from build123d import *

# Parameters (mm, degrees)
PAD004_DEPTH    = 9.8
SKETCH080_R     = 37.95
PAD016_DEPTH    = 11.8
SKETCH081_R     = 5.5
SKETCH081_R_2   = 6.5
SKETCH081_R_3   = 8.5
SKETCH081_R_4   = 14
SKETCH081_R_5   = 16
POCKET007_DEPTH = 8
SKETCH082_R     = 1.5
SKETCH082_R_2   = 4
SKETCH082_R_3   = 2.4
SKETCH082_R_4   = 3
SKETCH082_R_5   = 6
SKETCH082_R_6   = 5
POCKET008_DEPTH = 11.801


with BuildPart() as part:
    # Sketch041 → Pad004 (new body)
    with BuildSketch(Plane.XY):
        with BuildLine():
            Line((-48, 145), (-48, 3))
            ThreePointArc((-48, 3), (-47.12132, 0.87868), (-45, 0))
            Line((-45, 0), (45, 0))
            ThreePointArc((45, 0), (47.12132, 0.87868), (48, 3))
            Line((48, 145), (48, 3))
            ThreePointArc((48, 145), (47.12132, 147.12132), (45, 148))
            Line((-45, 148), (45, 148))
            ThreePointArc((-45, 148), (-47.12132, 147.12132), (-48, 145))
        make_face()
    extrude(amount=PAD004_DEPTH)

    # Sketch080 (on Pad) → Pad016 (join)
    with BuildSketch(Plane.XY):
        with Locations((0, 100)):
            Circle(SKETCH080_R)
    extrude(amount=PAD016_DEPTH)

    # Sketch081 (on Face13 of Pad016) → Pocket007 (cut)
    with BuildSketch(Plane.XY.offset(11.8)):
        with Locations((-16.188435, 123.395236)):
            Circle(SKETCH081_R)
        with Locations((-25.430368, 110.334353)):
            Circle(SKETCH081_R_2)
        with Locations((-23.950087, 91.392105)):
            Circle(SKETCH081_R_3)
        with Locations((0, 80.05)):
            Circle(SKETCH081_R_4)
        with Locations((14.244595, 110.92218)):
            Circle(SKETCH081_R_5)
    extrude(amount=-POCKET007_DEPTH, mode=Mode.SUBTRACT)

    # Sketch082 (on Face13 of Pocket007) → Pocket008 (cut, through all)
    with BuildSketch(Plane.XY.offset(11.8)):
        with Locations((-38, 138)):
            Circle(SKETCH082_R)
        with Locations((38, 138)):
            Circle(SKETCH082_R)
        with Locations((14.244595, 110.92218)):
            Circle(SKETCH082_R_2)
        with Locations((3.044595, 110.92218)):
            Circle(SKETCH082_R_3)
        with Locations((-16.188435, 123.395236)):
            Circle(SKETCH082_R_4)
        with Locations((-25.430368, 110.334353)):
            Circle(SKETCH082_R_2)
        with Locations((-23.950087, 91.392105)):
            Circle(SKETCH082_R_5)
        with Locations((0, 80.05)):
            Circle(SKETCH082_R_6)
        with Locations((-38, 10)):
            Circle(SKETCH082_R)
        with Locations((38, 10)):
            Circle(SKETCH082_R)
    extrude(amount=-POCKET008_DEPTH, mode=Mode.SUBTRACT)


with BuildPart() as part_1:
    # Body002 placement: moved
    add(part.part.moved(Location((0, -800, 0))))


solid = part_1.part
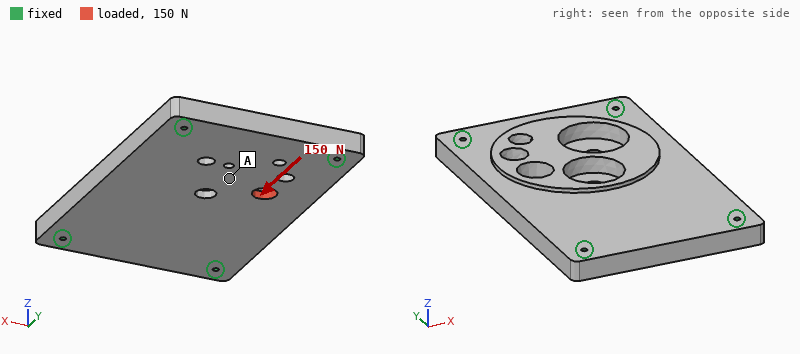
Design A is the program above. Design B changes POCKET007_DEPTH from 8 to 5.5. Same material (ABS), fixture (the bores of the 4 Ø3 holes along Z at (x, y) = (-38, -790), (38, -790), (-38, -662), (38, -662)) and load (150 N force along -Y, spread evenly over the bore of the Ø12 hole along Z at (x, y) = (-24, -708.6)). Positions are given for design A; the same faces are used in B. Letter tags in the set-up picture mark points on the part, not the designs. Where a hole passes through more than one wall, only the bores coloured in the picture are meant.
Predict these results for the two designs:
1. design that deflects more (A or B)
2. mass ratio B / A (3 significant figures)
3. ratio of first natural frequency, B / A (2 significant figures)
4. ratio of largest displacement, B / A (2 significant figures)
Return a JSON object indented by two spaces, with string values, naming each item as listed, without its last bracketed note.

{
  "design that deflects more": "A",
  "mass ratio B / A": "1.03",
  "ratio of first natural frequency, B / A": "0.98",
  "ratio of largest displacement, B / A": "0.76"
}
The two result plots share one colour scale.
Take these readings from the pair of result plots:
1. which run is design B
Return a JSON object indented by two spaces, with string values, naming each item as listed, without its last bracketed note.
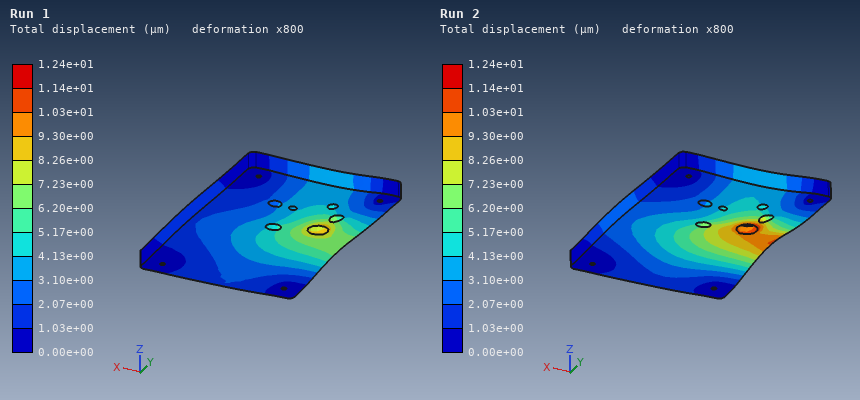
{
  "which run is design B": "Run 1"
}
